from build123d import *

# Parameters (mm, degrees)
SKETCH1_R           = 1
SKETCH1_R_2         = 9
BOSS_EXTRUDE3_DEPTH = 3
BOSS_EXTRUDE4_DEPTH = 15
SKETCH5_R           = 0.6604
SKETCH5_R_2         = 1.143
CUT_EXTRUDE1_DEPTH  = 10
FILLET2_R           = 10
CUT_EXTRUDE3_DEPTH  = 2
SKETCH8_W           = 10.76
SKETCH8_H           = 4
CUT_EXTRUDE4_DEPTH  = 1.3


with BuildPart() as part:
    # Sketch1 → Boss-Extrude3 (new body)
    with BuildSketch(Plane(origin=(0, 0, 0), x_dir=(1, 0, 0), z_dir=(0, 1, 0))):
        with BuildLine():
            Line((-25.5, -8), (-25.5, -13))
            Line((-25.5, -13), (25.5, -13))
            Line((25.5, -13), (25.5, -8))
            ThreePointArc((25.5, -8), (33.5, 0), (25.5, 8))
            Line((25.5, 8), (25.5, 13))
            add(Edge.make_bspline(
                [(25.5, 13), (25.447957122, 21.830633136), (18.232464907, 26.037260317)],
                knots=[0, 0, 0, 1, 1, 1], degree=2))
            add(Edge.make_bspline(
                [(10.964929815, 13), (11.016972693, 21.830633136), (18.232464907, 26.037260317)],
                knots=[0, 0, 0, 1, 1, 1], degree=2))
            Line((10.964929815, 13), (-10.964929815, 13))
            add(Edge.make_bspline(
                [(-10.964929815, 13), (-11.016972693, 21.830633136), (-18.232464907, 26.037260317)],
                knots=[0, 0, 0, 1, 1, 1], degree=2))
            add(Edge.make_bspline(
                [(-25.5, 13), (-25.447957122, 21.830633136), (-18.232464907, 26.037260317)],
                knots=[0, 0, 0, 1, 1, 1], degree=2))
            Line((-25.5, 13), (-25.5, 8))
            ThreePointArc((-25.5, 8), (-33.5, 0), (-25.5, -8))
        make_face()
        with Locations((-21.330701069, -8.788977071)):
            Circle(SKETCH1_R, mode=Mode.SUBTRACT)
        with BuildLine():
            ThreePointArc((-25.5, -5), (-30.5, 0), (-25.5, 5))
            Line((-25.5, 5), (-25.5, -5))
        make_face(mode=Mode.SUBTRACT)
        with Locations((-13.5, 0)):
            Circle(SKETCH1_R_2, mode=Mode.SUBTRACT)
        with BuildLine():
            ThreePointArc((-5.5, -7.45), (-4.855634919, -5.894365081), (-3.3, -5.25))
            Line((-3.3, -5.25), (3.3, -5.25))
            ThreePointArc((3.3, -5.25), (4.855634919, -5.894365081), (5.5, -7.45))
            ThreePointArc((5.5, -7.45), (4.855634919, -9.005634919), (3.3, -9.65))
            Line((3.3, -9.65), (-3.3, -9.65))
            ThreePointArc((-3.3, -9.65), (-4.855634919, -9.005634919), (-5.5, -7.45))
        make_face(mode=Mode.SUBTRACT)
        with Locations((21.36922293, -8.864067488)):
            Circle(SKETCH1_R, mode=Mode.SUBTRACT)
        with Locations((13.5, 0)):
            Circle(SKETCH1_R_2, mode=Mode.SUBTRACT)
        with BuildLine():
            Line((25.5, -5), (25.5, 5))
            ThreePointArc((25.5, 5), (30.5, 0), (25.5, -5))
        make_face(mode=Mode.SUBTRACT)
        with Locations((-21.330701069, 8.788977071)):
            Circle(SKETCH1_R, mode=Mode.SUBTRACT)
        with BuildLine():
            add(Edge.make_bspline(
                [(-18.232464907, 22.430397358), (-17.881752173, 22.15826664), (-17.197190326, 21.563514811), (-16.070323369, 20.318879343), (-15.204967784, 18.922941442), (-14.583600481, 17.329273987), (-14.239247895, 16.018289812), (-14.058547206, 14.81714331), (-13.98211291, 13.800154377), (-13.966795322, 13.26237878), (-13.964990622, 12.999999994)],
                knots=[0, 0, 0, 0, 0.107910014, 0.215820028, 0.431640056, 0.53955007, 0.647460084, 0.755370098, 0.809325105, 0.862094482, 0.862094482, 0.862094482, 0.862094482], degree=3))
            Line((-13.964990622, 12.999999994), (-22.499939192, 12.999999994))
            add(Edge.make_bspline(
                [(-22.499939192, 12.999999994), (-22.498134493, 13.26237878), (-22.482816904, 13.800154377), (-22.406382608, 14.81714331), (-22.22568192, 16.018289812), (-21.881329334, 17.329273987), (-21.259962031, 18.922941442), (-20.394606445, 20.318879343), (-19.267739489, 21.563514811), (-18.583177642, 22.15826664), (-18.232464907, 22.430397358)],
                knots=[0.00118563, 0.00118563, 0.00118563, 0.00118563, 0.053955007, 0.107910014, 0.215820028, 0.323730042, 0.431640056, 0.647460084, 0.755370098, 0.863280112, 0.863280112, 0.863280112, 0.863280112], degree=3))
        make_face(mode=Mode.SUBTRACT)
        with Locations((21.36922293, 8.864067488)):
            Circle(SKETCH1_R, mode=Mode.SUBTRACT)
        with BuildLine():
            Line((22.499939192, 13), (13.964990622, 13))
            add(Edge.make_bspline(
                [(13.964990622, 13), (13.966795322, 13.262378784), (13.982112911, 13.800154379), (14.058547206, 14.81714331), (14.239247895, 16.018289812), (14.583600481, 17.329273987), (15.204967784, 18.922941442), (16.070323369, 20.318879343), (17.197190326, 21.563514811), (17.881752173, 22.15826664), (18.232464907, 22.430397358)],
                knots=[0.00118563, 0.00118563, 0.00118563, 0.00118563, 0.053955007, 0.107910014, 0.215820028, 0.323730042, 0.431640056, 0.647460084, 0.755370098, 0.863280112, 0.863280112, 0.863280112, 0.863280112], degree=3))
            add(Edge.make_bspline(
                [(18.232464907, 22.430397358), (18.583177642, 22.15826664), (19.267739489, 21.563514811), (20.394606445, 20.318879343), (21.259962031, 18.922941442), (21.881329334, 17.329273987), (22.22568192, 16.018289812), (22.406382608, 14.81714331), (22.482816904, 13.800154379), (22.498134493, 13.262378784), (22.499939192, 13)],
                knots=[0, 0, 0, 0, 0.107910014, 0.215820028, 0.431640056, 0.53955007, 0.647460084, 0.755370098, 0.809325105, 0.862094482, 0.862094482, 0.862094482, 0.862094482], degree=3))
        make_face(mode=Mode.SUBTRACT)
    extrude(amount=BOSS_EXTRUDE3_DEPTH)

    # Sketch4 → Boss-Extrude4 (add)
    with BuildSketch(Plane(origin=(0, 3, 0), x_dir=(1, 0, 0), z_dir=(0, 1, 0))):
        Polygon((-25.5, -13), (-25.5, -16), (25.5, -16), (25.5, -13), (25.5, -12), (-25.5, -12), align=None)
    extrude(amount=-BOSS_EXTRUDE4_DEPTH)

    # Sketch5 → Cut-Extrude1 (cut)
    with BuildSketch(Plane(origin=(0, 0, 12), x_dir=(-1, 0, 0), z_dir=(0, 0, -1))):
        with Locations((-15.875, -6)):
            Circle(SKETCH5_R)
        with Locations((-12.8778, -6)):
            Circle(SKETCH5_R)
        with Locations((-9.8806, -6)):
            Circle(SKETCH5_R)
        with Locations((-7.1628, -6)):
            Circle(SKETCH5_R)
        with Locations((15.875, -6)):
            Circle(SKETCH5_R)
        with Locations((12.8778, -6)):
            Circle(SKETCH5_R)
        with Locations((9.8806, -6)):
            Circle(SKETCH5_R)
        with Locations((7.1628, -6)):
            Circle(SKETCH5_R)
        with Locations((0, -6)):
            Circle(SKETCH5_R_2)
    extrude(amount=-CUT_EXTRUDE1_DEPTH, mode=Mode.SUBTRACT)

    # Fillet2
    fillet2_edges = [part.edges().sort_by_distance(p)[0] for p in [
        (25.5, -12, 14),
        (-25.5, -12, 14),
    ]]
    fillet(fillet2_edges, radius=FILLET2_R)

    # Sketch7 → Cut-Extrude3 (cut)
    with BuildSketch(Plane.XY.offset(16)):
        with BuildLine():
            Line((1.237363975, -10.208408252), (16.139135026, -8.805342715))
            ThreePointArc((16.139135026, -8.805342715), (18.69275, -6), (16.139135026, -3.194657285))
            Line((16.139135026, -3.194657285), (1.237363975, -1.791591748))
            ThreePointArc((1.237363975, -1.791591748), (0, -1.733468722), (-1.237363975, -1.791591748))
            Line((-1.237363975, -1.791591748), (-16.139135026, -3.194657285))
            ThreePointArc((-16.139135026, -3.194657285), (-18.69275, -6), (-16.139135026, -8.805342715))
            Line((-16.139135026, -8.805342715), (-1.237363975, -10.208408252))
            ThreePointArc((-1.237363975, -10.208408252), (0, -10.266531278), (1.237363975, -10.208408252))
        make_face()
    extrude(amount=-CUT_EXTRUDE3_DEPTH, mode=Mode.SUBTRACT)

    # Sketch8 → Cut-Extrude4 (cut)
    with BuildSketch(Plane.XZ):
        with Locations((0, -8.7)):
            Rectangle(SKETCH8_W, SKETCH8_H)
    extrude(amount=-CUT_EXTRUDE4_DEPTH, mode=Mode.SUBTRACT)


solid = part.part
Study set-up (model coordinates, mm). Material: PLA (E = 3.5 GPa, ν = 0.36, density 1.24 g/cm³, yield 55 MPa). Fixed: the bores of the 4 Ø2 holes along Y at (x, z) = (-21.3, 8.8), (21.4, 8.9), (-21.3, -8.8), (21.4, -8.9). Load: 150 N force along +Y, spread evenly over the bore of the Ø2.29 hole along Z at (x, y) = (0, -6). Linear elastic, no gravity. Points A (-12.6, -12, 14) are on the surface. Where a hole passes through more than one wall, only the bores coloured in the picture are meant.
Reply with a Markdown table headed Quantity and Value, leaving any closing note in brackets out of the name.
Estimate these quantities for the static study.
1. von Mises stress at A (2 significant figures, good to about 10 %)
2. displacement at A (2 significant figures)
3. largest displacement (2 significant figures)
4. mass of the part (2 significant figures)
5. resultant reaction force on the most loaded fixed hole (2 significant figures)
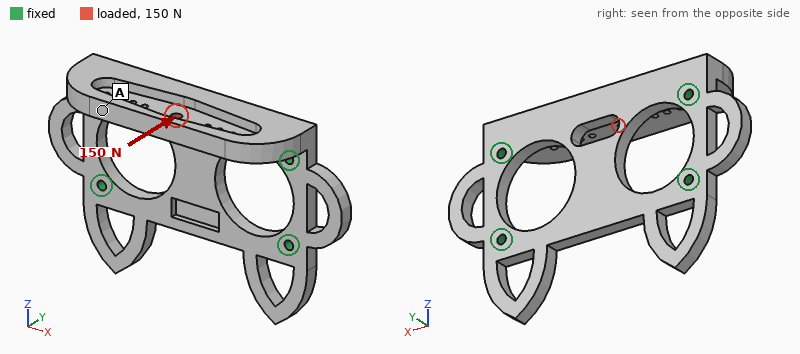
| Quantity | Value |
|---|---|
| von Mises stress at A | 2.7 MPa |
| displacement at A | 0.17 mm |
| largest displacement | 0.22 mm |
| mass of the part | 6.5 g |
| resultant reaction force on the most loaded fixed hole | 86 N |
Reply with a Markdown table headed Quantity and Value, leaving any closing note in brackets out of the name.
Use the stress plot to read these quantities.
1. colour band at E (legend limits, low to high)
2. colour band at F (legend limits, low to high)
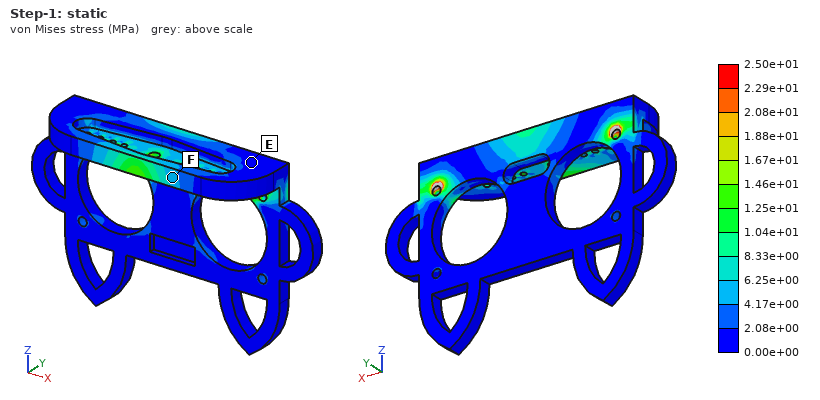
| Quantity | Value |
|---|---|
| colour band at E | 0.00e+00 to 2.08e+00 MPa |
| colour band at F | 4.17e+00 to 6.25e+00 MPa |
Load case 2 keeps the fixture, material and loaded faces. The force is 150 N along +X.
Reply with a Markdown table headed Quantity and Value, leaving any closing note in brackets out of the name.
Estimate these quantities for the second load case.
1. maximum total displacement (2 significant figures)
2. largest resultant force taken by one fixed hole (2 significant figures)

| Quantity | Value |
|---|---|
| maximum total displacement | 45 µm |
| largest resultant force taken by one fixed hole | 76 N |
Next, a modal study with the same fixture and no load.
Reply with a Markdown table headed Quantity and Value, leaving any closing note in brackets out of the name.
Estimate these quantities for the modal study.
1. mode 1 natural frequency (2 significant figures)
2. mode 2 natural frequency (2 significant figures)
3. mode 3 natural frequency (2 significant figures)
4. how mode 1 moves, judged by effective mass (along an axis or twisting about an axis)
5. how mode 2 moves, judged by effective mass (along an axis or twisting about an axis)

| Quantity | Value |
|---|---|
| mode 1 natural frequency | 2000 Hz |
| mode 2 natural frequency | 2500 Hz |
| mode 3 natural frequency | 2900 Hz |
| how mode 1 moves, judged by effective mass | along Z |
| how mode 2 moves, judged by effective mass | along Y |
